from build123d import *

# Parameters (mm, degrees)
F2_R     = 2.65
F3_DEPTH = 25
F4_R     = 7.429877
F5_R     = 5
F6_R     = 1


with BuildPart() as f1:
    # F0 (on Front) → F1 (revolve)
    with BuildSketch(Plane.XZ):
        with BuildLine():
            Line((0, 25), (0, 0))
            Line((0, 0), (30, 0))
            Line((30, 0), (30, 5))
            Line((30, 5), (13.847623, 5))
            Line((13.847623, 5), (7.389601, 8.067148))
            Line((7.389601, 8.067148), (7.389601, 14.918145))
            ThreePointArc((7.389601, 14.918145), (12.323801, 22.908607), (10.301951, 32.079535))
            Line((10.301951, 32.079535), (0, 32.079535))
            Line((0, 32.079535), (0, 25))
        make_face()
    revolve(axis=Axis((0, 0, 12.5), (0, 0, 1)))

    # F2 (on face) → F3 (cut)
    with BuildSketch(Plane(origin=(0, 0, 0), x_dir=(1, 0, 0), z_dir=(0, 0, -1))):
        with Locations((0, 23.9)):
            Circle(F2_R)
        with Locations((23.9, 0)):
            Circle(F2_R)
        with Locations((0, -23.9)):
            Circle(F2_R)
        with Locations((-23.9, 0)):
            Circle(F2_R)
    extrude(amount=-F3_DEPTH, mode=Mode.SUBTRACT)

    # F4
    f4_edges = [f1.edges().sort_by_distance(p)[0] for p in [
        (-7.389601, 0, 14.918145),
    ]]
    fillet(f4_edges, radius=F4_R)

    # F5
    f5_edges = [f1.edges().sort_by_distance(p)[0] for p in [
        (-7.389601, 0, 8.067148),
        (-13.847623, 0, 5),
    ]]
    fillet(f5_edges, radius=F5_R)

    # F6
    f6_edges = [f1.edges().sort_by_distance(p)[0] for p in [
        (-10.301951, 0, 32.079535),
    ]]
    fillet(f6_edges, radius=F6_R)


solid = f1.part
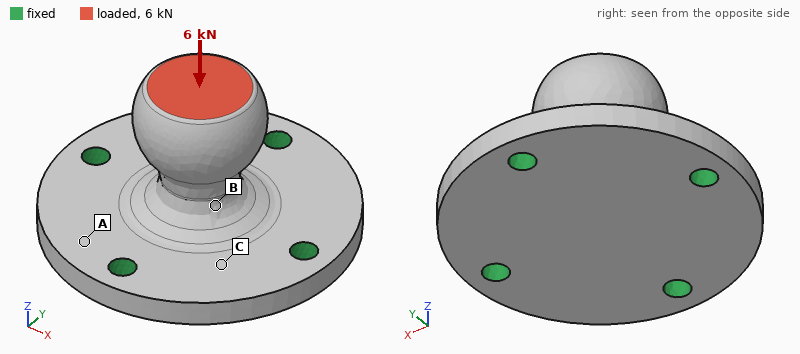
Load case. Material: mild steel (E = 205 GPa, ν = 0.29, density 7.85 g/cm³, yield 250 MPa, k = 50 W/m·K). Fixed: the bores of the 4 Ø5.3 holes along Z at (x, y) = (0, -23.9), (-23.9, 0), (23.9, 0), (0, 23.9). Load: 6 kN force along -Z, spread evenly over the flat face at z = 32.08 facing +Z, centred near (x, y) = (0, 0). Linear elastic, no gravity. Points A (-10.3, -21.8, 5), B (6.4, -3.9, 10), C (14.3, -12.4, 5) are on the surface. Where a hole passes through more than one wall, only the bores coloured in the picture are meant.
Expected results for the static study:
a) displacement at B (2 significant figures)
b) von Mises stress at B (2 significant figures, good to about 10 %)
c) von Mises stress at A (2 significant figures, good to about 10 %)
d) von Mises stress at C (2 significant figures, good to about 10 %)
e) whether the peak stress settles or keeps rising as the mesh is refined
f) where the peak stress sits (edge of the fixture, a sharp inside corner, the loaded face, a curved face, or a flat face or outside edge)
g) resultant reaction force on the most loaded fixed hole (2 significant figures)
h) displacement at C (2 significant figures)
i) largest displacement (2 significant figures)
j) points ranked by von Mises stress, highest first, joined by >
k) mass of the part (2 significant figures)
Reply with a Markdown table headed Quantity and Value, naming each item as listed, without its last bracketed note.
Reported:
| Quantity | Value |
|---|---|
| displacement at B | 13 µm |
| von Mises stress at B | 62 MPa |
| von Mises stress at A | 20 MPa |
| von Mises stress at C | 31 MPa |
| whether the peak stress settles or keeps rising as the mesh is refined | keeps rising |
| where the peak stress sits | edge of the fixture |
| resultant reaction force on the most loaded fixed hole | 1.6 kN |
| displacement at C | 5.4 µm |
| largest displacement | 15 µm |
| points ranked by von Mises stress, highest first, joined by > | B > C > A |
| mass of the part | 180 g |
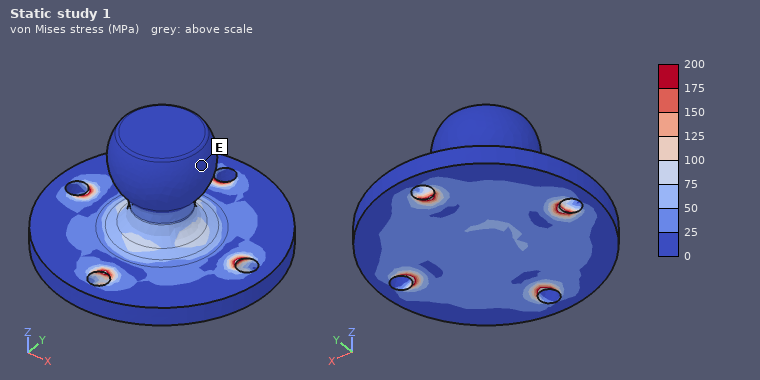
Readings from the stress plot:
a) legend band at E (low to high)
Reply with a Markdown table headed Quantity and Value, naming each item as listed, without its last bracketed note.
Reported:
| Quantity | Value |
|---|---|
| legend band at E | 0 to 25 MPa |
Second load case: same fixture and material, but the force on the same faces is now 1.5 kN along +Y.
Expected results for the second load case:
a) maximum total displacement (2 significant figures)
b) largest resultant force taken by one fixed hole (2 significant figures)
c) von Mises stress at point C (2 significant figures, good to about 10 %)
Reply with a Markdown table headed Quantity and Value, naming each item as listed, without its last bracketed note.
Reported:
| Quantity | Value |
|---|---|
| maximum total displacement | 33 µm |
| largest resultant force taken by one fixed hole | 1.2 kN |
| von Mises stress at point C | 17 MPa |
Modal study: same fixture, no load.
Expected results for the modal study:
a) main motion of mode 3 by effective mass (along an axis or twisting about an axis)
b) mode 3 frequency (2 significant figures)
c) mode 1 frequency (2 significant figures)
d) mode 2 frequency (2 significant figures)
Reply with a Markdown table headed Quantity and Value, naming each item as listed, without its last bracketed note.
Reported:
| Quantity | Value |
|---|---|
| main motion of mode 3 by effective mass | along Z |
| mode 3 frequency | 11 kHz |
| mode 1 frequency | 6300 Hz |
| mode 2 frequency | 6300 Hz |
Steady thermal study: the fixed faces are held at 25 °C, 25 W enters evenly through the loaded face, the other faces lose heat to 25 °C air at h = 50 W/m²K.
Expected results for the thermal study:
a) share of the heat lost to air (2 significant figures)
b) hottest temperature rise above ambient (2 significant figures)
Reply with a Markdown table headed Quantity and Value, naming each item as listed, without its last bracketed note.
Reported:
| Quantity | Value |
|---|---|
| share of the heat lost to air | 23 % |
| hottest temperature rise above ambient | 62 K |
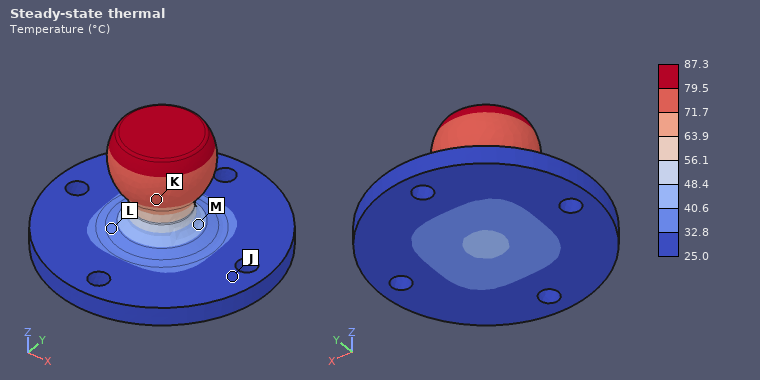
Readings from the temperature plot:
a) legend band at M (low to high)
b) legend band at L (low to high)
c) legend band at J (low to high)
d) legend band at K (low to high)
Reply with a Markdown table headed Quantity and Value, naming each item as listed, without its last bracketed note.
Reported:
| Quantity | Value |
|---|---|
| legend band at M | 40.6 to 48.4 °C |
| legend band at L | 32.8 to 40.6 °C |
| legend band at J | 25.0 to 32.8 °C |
| legend band at K | 71.7 to 79.5 °C |
